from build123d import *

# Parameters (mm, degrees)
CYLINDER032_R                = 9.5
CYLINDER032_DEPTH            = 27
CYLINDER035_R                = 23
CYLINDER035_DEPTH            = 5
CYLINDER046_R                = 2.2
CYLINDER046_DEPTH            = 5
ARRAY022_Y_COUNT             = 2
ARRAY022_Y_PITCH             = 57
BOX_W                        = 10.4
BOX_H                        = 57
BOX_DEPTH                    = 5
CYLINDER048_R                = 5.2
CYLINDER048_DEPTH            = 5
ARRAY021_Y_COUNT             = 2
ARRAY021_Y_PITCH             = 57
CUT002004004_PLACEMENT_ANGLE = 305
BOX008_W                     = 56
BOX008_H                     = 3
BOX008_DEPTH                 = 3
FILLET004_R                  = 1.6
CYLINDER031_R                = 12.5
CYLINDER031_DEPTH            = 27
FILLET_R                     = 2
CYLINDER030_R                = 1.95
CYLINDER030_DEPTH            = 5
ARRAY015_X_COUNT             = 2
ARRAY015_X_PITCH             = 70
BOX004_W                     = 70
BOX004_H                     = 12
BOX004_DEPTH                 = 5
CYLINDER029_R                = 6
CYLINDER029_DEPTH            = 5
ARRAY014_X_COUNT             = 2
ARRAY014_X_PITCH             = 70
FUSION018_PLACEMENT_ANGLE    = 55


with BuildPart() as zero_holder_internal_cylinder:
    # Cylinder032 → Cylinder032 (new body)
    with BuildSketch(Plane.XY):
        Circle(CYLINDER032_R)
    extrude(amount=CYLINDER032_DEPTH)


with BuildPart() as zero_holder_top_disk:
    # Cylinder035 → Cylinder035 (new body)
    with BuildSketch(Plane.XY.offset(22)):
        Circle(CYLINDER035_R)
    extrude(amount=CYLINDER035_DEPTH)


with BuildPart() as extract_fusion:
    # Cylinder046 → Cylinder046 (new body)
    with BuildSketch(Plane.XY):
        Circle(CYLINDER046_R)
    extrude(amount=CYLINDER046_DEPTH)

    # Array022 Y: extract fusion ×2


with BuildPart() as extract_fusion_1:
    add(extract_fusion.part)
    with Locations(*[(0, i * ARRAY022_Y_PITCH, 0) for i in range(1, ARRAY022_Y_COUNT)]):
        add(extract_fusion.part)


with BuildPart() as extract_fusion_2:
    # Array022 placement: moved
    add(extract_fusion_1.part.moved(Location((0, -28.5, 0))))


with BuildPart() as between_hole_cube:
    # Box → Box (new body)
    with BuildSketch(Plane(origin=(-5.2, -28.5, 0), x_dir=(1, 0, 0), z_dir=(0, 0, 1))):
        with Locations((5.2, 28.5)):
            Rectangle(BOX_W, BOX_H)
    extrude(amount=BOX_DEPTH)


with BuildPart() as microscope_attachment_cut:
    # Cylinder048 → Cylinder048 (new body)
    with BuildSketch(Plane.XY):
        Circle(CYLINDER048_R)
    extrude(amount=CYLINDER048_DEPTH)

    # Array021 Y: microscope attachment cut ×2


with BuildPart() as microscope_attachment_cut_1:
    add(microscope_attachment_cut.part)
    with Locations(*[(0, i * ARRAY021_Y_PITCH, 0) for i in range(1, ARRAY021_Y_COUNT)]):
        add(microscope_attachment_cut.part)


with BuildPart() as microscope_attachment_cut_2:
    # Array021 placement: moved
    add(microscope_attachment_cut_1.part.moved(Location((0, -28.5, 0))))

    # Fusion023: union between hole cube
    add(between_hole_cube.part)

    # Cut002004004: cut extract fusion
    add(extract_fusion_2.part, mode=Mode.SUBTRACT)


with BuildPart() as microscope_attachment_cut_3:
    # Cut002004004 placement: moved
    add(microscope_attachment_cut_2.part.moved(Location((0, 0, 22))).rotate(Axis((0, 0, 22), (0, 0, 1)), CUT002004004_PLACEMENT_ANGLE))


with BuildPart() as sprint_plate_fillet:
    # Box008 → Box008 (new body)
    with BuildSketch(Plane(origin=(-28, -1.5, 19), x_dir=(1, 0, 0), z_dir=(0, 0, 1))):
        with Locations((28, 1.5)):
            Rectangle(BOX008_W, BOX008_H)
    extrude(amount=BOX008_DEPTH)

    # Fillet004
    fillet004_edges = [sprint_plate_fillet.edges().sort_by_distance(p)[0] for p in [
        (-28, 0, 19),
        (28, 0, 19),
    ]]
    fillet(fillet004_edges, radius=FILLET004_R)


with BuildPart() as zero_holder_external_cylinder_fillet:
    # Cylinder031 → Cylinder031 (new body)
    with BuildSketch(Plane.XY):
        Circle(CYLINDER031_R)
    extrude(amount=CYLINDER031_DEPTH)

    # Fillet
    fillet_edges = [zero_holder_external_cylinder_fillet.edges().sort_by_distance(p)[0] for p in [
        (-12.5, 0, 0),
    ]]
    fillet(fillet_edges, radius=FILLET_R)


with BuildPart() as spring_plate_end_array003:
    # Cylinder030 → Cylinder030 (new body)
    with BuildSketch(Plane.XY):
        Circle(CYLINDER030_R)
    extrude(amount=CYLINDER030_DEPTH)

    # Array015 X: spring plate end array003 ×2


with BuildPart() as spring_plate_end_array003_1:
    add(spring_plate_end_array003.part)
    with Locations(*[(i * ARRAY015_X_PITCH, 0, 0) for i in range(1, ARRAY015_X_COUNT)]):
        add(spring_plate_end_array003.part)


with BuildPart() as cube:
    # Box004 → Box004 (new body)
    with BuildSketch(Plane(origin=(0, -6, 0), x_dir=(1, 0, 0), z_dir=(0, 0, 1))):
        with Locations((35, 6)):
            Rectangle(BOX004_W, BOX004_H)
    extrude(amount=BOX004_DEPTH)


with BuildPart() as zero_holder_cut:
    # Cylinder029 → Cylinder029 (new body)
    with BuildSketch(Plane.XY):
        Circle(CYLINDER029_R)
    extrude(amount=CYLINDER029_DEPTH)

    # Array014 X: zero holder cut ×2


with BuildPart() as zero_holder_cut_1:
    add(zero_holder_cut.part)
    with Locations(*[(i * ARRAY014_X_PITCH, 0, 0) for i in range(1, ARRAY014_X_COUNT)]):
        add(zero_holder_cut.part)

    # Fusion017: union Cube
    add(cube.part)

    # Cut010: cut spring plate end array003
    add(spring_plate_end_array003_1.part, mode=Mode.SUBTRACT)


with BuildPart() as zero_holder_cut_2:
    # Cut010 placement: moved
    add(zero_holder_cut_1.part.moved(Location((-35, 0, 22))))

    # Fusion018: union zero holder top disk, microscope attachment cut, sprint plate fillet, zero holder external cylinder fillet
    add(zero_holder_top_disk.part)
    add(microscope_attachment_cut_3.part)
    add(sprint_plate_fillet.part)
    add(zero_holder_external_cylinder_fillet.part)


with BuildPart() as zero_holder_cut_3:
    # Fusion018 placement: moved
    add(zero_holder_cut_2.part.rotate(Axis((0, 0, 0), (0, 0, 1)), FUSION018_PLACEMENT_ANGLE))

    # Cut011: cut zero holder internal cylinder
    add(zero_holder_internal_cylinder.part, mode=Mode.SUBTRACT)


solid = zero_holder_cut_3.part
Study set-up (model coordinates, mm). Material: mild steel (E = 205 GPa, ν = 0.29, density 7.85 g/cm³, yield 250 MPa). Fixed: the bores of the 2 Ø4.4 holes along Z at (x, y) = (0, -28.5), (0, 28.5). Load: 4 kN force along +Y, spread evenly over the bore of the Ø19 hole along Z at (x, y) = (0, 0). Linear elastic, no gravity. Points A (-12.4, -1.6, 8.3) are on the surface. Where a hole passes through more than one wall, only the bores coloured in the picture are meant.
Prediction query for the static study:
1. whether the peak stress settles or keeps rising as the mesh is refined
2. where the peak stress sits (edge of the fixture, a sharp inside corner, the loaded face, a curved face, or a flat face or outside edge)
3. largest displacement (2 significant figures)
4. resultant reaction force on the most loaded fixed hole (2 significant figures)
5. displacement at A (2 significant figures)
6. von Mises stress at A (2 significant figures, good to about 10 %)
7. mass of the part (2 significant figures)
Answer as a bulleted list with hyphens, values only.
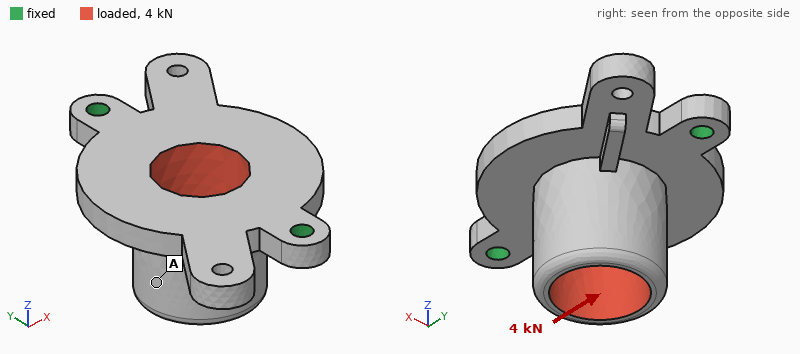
- keeps rising
- edge of the fixture
- 31 µm
- 2.2 kN
- 20 µm
- 20 MPa
- 110 g
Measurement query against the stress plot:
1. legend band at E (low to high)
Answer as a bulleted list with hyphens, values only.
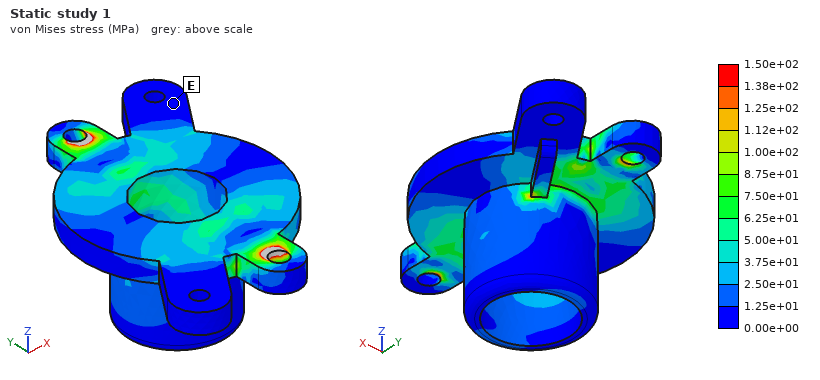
- 0.00e+00 to 1.25e+01 MPa
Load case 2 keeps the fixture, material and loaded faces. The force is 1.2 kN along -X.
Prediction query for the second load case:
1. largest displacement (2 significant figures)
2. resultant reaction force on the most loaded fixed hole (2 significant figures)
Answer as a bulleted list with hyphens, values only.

- 71 µm
- 600 N
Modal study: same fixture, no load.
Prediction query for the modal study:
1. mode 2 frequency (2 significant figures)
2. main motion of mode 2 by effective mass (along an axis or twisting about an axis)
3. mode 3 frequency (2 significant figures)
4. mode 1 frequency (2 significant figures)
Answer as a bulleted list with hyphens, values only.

- 5100 Hz
- along Z
- 7100 Hz
- 2500 Hz
